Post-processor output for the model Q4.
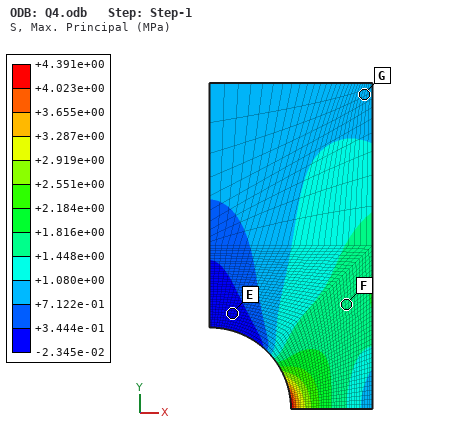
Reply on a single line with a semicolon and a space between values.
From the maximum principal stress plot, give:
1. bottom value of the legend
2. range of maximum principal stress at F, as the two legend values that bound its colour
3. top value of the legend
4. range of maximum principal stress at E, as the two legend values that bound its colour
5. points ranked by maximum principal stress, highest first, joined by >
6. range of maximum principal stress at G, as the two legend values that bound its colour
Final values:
-2.345e-02 MPa; +1.448e+00 to +1.816e+00 MPa; +4.391e+00 MPa; -2.345e-02 to +3.444e-01 MPa; F > G > E; +7.122e-01 to +1.080e+00 MPa
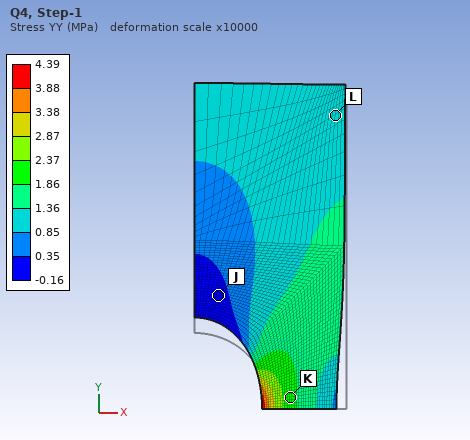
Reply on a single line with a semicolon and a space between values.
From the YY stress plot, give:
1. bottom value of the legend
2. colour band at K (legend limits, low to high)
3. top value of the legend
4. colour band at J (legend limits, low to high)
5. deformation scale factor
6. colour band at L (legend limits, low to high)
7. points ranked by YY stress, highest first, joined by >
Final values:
-0.16 MPa; 1.86 to 2.37 MPa; 4.39 MPa; -0.16 to 0.35 MPa; 10000; 0.85 to 1.36 MPa; K > L > J
